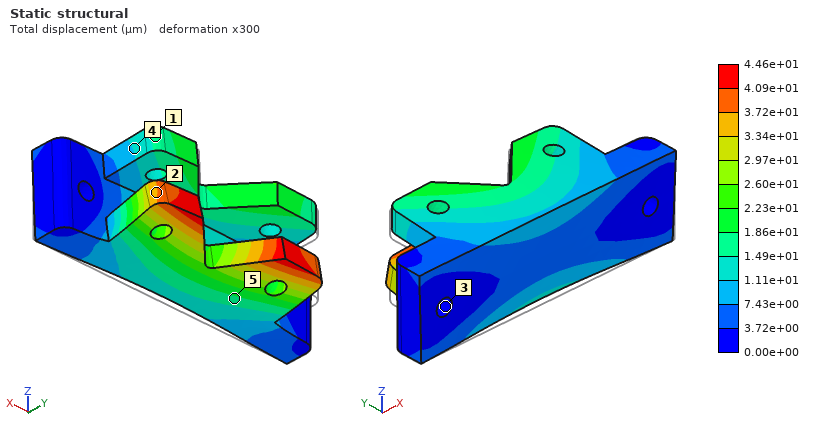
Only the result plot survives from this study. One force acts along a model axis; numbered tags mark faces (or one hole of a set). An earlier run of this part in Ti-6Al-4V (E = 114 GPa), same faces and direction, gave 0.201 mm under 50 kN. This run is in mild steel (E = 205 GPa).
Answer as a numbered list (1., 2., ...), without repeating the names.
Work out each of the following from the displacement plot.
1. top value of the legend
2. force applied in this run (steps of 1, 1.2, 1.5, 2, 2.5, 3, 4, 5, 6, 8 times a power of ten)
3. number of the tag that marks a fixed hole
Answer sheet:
1. 4.46e+01 µm
2. 20 kN
3. 3
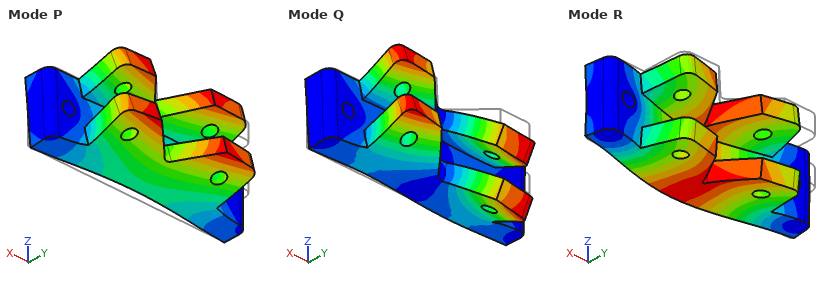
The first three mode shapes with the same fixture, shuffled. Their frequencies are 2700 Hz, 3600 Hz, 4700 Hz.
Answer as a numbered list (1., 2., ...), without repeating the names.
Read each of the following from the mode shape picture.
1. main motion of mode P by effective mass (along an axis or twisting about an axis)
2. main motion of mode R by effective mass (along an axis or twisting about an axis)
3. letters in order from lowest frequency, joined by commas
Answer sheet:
1. along Z
2. along Y
3. P, R, Q
